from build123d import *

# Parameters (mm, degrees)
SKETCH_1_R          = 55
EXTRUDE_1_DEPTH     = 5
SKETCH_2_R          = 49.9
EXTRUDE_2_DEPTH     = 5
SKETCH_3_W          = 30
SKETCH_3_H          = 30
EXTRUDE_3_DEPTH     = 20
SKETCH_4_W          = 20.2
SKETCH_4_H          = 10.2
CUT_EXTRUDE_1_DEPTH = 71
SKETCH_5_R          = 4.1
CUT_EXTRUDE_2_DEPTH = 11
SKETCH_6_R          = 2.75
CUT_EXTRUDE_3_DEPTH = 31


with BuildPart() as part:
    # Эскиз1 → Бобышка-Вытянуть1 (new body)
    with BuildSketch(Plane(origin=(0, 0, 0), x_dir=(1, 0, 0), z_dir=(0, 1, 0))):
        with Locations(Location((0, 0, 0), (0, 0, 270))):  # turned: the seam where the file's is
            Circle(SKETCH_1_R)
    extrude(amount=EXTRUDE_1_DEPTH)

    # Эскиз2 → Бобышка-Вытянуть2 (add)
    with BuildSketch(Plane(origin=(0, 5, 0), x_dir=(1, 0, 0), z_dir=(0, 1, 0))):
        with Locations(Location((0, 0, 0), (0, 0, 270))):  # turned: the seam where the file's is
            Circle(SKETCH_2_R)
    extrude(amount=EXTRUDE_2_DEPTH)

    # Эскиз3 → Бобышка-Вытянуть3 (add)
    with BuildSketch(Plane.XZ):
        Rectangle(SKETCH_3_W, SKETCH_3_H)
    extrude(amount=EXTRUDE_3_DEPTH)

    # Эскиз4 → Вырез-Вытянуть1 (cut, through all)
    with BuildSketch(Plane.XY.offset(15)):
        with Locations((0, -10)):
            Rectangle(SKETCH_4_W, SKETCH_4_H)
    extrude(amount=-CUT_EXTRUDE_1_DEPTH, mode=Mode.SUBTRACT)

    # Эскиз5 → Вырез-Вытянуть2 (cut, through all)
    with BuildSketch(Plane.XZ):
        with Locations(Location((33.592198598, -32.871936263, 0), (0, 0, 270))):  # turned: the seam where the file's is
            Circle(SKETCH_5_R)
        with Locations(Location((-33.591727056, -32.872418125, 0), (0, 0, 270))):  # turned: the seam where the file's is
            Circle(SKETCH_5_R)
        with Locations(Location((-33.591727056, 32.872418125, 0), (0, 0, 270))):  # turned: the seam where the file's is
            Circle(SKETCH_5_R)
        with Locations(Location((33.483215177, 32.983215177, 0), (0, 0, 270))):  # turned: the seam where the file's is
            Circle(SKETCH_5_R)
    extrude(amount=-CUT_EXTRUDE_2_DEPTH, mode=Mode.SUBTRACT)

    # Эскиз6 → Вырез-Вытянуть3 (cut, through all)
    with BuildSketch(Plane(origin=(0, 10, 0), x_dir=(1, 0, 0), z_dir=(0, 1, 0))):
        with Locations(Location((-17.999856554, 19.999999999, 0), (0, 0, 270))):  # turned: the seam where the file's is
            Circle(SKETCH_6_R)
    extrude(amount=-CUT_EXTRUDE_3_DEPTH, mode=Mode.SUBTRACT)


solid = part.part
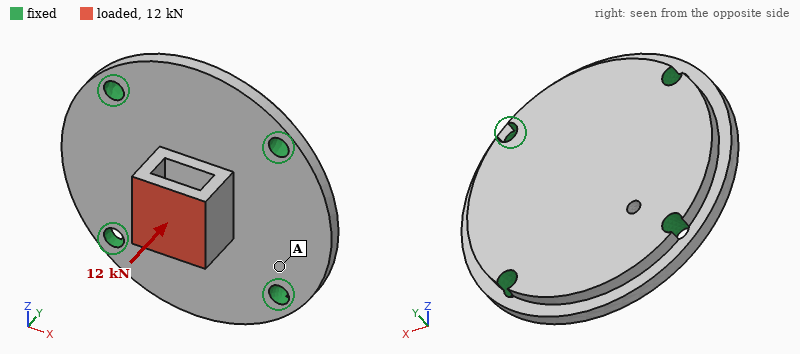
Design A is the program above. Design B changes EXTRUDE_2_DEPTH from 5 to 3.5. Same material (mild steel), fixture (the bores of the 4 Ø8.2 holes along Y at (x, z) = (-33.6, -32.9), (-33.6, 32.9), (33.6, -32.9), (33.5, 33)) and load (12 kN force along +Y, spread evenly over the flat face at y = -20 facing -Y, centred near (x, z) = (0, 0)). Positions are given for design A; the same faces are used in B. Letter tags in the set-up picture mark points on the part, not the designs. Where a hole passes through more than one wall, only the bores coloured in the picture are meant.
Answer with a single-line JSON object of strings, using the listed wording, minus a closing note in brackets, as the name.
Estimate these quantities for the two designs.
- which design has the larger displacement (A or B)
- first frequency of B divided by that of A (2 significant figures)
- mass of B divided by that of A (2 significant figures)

{"which design has the larger displacement": "B", "first frequency of B divided by that of A": "0.88", "mass of B divided by that of A": "0.88"}
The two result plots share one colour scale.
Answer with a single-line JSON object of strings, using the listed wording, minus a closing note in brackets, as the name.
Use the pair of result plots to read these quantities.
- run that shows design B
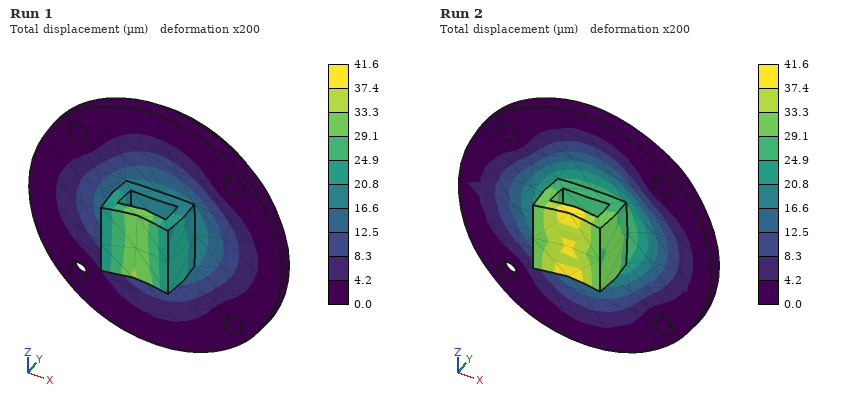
{"run that shows design B": "Run 2"}
